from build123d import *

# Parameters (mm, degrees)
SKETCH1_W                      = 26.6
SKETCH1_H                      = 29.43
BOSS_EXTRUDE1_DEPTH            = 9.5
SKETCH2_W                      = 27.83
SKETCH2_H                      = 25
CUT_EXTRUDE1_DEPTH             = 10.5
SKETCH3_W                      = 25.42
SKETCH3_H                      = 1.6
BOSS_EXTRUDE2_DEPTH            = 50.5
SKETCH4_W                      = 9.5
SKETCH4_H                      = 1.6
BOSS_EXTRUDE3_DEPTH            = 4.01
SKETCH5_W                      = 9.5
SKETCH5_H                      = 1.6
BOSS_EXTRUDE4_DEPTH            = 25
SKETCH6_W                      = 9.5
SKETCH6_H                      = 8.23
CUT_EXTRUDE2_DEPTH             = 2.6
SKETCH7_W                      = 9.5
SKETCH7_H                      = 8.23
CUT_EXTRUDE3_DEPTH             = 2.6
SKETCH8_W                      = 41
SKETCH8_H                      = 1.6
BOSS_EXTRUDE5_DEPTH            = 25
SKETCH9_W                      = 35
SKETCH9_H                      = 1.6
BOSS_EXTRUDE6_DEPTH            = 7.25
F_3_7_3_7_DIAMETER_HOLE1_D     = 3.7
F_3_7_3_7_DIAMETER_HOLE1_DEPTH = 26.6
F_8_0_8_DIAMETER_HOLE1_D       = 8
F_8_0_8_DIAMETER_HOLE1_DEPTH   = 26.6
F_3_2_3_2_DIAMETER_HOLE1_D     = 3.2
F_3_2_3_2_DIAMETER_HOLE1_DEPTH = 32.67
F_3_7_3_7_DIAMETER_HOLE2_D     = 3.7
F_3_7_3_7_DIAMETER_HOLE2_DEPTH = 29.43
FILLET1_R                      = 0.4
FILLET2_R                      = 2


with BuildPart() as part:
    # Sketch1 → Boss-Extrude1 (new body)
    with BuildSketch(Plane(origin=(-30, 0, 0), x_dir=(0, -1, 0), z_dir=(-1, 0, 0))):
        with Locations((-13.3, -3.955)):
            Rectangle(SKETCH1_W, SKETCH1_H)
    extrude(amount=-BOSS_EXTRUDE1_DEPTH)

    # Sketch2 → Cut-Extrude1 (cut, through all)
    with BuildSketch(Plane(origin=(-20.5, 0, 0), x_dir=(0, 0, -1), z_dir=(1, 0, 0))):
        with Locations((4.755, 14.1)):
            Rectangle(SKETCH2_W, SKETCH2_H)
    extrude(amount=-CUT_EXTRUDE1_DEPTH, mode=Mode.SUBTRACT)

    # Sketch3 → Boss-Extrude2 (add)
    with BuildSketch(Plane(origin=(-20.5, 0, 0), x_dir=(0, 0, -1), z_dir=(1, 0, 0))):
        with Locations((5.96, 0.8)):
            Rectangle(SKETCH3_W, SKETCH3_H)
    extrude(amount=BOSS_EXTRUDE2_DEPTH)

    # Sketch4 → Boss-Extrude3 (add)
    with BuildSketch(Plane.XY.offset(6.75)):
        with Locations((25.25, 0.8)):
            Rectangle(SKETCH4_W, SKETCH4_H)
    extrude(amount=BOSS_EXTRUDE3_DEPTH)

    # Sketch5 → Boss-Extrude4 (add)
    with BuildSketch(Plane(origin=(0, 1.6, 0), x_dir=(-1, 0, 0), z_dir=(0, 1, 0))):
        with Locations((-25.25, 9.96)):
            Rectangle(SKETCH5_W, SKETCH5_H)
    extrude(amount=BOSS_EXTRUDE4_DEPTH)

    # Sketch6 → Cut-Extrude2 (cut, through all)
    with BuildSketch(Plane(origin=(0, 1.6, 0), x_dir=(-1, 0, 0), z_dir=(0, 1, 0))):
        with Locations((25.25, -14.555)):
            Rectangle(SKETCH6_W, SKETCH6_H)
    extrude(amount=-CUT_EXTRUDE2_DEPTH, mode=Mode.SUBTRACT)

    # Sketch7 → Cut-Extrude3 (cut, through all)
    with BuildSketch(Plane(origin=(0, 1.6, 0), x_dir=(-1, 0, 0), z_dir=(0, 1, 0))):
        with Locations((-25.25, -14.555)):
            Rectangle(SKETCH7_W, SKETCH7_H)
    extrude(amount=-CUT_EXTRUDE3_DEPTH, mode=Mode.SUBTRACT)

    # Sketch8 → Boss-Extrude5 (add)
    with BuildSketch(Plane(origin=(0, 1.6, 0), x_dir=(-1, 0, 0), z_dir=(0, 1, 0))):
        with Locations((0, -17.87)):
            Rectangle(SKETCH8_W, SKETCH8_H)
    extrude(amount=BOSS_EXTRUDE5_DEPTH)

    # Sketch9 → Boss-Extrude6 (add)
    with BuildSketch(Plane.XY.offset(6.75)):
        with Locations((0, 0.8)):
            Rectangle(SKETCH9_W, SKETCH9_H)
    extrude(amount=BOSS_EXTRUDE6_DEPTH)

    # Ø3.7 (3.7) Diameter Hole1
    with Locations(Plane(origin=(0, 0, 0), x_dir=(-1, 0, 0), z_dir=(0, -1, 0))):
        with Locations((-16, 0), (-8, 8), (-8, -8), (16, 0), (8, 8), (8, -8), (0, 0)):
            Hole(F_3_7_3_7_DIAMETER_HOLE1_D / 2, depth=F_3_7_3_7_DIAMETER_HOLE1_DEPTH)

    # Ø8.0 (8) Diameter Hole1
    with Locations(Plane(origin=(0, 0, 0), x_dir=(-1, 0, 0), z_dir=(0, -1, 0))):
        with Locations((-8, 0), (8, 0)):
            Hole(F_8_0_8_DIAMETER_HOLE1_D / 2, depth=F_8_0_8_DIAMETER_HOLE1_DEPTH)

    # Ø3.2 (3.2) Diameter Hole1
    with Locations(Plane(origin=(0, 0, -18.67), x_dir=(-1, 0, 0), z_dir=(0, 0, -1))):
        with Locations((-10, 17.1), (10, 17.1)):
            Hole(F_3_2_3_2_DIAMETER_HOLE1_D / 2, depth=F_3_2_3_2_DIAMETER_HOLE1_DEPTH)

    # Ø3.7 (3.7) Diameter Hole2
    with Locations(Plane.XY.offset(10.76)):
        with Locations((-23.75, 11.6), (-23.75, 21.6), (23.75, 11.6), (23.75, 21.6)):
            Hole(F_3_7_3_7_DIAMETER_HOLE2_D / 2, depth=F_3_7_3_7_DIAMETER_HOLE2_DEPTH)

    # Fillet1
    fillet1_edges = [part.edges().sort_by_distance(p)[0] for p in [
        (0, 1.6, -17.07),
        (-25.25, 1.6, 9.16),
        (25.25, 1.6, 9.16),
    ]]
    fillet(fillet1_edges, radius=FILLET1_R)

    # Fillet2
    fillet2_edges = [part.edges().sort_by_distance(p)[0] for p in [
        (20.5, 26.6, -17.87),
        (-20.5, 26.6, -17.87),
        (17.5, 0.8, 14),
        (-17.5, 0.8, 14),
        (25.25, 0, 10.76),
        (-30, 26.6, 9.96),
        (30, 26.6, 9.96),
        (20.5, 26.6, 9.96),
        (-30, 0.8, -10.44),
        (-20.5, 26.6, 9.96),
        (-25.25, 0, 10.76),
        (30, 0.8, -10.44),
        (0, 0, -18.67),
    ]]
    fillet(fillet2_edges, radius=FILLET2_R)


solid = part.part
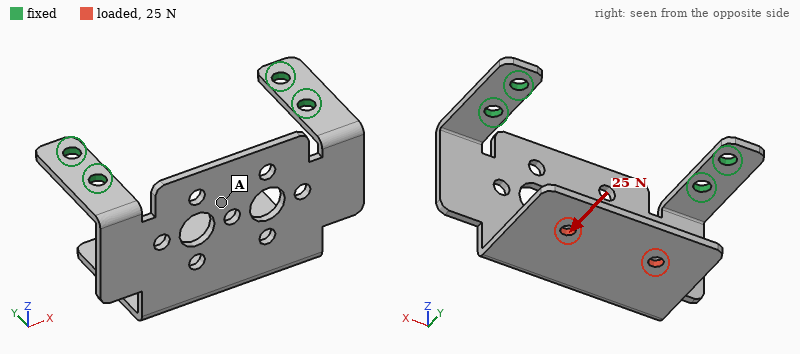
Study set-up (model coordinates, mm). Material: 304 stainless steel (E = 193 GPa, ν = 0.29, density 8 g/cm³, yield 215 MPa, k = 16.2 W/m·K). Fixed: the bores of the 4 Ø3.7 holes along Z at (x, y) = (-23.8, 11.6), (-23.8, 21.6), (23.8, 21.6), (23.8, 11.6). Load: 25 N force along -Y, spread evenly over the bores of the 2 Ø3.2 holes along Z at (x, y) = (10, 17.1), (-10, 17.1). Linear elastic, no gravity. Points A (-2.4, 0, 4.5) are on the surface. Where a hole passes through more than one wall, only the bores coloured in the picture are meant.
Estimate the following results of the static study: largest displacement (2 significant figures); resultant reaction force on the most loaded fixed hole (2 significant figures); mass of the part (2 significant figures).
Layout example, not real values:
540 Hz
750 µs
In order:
0.36 mm
12 N
37 g
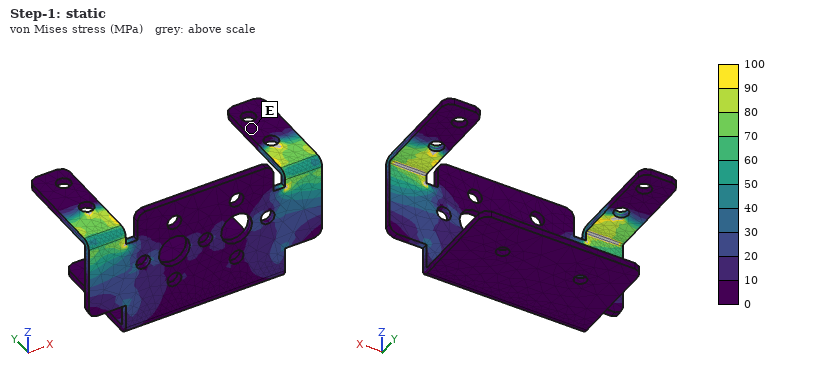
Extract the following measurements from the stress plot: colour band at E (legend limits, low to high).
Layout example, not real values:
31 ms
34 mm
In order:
0 to 10 MPa
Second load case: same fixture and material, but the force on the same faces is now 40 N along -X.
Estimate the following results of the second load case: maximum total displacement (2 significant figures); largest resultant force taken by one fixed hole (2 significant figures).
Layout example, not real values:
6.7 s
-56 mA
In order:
0.11 mm
39 N
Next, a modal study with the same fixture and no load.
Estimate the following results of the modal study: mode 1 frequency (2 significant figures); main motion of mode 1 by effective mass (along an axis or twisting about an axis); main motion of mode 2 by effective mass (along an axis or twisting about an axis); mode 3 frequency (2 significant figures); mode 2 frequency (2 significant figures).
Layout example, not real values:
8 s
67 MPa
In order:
340 Hz
along Y
along X
1100 Hz
910 Hz
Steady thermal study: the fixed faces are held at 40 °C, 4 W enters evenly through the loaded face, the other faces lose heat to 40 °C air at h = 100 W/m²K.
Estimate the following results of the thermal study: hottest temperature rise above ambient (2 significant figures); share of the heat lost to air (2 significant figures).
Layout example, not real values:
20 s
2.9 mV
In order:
35 K
100 %
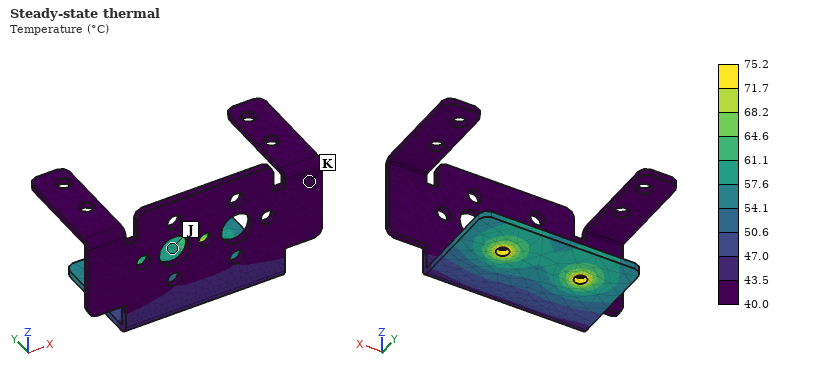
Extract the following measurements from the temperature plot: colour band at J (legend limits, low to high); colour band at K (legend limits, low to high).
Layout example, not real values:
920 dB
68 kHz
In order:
57.6 to 61.1 °C
40.0 to 43.5 °C
